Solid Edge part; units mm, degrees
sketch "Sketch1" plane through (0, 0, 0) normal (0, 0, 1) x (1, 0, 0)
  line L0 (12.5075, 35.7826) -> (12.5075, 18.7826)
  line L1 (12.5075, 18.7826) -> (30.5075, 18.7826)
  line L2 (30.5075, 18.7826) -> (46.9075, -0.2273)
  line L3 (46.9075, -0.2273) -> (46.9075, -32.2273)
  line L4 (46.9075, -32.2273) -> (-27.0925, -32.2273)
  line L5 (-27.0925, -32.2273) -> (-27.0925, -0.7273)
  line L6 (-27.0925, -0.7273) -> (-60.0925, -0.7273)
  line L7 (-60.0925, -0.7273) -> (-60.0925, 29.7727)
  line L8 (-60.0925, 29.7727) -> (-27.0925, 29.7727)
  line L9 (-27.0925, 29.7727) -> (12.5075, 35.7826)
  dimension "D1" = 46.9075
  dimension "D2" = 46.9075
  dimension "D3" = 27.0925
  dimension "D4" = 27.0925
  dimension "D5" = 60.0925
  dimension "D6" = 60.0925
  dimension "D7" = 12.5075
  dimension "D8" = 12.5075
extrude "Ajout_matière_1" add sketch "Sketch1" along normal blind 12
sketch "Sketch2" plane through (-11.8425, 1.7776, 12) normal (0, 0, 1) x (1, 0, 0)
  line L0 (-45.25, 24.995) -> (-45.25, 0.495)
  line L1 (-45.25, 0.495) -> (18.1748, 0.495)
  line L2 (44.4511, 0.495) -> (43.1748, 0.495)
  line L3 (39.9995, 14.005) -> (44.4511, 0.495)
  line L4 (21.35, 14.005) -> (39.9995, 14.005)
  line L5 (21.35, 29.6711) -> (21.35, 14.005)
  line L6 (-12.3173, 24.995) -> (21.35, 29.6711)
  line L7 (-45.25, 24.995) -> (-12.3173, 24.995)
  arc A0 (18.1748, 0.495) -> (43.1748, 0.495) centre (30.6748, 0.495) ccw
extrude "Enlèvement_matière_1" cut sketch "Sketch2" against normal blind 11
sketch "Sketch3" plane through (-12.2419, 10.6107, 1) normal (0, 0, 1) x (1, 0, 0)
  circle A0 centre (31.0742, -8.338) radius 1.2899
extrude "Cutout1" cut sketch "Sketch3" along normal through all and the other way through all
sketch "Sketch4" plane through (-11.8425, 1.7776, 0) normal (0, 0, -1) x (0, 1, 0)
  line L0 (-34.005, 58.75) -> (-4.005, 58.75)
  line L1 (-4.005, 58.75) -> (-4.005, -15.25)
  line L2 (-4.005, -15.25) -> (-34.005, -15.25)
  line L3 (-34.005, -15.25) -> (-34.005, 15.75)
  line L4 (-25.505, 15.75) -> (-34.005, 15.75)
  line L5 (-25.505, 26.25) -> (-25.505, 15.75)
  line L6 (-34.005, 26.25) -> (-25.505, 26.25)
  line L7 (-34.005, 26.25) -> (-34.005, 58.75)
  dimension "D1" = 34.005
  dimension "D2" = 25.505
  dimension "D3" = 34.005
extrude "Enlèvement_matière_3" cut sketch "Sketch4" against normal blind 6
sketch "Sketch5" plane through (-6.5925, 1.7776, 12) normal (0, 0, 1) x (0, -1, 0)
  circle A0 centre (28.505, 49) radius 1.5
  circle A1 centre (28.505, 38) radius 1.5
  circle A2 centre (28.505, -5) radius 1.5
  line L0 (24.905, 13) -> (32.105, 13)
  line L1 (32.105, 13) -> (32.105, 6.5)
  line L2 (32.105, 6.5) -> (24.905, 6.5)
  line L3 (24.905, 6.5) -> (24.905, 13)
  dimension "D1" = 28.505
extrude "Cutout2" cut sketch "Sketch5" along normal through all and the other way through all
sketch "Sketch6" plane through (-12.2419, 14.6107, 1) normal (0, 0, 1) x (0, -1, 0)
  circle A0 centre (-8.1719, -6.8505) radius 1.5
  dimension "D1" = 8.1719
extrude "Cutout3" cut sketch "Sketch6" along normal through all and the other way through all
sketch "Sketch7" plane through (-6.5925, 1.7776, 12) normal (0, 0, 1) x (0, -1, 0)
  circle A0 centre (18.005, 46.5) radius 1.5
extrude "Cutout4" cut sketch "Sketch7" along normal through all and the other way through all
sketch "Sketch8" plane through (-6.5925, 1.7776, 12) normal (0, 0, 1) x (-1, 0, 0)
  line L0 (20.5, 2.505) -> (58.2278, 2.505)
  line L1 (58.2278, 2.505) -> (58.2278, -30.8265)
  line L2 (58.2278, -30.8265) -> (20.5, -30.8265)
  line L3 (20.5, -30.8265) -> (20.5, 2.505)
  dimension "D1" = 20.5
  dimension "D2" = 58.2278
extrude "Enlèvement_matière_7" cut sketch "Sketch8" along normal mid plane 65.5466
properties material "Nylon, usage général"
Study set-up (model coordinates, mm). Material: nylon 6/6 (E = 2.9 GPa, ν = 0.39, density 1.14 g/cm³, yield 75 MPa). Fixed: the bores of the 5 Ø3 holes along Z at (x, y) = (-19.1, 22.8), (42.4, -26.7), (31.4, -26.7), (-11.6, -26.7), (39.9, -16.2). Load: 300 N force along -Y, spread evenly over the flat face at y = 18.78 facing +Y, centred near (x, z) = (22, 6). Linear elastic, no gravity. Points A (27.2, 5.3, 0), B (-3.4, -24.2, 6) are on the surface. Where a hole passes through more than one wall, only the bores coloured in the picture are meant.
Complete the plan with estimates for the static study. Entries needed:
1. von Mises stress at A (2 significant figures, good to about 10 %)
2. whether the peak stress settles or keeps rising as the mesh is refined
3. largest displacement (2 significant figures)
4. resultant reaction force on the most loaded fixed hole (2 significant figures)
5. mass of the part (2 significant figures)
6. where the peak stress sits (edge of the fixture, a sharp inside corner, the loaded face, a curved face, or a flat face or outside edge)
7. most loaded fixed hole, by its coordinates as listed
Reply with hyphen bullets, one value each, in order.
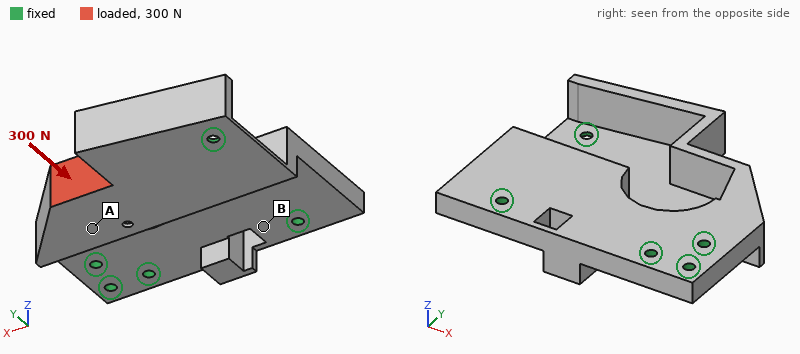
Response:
- 7.7 MPa
- keeps rising
- 1.2 mm
- 130 N
- 24 g
- edge of the fixture
- (39.9, -16.2)
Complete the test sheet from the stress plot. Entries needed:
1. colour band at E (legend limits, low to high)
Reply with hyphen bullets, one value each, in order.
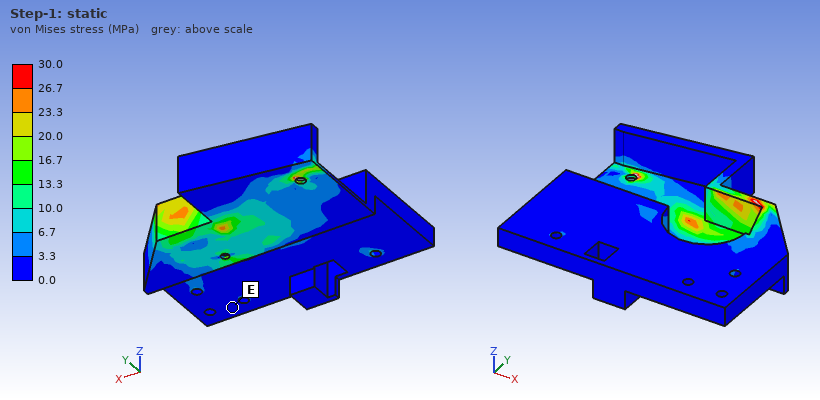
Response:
- 0.0 to 3.3 MPa
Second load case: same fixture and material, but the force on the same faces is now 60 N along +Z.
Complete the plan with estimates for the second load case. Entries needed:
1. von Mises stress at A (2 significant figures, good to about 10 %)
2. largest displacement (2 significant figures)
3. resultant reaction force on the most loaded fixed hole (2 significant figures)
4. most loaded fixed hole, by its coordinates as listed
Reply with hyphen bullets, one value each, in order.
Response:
- 3.1 MPa
- 0.92 mm
- 97 N
- (39.9, -16.2)
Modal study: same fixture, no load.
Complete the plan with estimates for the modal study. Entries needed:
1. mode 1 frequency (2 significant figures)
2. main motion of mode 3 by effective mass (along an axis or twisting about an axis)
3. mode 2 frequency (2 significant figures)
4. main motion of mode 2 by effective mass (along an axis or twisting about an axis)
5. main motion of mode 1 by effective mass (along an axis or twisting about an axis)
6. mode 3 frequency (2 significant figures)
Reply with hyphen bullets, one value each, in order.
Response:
- 650 Hz
- along Z
- 1300 Hz
- along Z
- along Z
- 1700 Hz
